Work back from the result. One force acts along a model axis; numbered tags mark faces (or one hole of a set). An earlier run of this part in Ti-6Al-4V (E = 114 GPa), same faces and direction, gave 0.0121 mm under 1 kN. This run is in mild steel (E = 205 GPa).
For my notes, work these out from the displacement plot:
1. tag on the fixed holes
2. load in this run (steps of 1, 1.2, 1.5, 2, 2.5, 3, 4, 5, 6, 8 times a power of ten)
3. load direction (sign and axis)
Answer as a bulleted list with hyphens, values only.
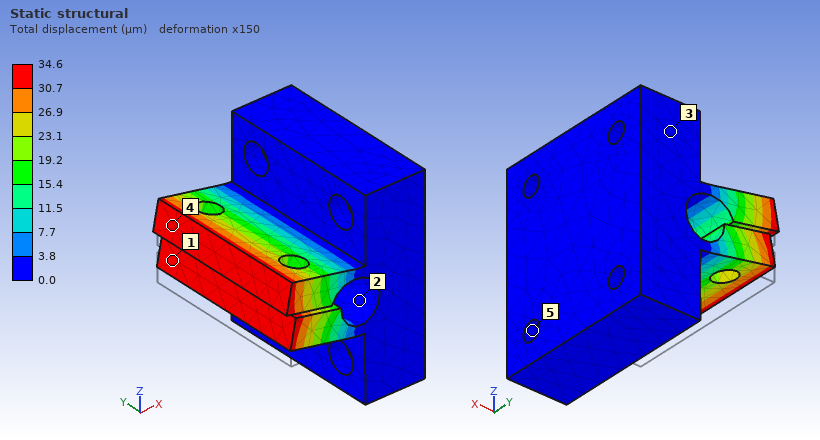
- 5
- 5 kN
- +Z
